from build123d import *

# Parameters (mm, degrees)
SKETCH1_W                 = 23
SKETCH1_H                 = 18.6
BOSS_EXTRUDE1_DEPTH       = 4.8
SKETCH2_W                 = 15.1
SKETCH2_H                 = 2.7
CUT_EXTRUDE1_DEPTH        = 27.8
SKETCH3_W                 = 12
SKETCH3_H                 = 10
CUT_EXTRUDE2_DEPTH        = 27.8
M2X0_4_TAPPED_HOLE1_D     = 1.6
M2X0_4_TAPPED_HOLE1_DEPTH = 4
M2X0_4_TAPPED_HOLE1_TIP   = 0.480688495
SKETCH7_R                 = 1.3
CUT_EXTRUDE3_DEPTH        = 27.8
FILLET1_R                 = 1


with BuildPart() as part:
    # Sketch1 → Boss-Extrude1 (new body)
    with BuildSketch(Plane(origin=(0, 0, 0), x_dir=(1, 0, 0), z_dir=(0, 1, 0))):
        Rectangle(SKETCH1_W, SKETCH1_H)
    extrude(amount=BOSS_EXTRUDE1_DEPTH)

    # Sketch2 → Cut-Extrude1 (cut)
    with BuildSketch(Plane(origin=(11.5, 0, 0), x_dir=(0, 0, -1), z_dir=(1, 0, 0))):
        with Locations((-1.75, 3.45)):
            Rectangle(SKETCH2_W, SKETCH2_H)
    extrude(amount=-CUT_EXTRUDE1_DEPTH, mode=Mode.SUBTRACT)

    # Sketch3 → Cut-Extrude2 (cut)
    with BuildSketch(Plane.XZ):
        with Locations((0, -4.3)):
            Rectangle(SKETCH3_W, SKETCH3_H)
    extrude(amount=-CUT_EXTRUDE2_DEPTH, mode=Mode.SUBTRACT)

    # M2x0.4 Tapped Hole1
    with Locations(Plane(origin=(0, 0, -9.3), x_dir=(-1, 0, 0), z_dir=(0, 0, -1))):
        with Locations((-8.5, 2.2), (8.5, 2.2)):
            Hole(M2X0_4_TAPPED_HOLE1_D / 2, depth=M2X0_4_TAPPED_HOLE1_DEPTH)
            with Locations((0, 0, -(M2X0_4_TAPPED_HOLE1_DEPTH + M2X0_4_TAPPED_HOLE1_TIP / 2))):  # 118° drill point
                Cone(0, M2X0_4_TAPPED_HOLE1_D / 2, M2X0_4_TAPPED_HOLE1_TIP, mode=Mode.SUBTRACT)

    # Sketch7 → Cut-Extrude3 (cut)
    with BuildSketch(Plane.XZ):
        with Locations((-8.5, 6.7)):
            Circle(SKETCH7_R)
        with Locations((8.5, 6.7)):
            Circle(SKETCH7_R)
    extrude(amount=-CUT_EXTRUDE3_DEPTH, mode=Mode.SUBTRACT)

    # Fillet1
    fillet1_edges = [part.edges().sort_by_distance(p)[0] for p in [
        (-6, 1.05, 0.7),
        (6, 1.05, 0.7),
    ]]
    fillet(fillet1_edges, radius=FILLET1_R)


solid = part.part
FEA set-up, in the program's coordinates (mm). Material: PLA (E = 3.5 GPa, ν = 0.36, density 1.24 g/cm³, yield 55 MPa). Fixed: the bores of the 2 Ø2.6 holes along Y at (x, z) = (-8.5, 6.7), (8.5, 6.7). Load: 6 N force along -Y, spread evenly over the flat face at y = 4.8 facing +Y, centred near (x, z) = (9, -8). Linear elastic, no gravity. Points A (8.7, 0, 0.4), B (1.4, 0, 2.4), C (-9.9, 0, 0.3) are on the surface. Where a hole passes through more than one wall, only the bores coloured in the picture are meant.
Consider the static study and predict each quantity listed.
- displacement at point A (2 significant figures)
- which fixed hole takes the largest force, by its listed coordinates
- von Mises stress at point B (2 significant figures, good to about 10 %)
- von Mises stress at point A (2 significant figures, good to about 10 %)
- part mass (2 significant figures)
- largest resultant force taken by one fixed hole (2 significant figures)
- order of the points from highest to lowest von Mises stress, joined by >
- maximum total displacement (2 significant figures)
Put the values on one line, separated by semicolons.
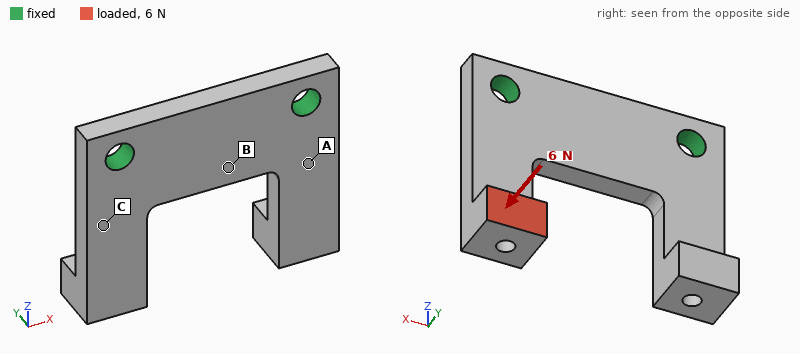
0.056 mm; (8.5, 6.7); 3.2 MPa; 11 MPa; 0.89 g; 6.6 N; A > B > C; 0.34 mm
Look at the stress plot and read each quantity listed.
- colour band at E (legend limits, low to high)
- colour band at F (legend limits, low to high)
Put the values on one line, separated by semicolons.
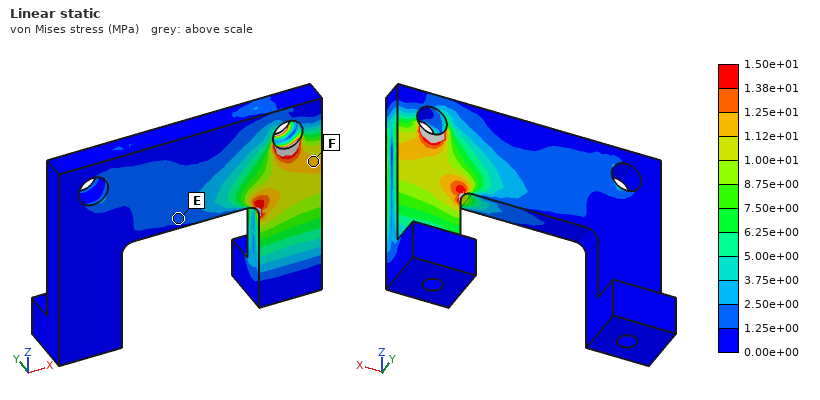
1.25e+00 to 2.50e+00 MPa; 1.12e+01 to 1.25e+01 MPa
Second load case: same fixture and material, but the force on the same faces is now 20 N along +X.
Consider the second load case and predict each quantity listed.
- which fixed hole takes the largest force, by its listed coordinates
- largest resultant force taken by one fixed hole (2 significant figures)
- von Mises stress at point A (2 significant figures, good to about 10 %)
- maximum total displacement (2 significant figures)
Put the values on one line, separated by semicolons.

(-8.5, 6.7); 23 N; 16 MPa; 0.33 mm
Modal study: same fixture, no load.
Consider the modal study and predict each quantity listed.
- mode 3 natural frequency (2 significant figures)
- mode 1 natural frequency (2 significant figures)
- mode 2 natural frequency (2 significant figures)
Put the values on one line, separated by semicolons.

5200 Hz; 2000 Hz; 2100 Hz
